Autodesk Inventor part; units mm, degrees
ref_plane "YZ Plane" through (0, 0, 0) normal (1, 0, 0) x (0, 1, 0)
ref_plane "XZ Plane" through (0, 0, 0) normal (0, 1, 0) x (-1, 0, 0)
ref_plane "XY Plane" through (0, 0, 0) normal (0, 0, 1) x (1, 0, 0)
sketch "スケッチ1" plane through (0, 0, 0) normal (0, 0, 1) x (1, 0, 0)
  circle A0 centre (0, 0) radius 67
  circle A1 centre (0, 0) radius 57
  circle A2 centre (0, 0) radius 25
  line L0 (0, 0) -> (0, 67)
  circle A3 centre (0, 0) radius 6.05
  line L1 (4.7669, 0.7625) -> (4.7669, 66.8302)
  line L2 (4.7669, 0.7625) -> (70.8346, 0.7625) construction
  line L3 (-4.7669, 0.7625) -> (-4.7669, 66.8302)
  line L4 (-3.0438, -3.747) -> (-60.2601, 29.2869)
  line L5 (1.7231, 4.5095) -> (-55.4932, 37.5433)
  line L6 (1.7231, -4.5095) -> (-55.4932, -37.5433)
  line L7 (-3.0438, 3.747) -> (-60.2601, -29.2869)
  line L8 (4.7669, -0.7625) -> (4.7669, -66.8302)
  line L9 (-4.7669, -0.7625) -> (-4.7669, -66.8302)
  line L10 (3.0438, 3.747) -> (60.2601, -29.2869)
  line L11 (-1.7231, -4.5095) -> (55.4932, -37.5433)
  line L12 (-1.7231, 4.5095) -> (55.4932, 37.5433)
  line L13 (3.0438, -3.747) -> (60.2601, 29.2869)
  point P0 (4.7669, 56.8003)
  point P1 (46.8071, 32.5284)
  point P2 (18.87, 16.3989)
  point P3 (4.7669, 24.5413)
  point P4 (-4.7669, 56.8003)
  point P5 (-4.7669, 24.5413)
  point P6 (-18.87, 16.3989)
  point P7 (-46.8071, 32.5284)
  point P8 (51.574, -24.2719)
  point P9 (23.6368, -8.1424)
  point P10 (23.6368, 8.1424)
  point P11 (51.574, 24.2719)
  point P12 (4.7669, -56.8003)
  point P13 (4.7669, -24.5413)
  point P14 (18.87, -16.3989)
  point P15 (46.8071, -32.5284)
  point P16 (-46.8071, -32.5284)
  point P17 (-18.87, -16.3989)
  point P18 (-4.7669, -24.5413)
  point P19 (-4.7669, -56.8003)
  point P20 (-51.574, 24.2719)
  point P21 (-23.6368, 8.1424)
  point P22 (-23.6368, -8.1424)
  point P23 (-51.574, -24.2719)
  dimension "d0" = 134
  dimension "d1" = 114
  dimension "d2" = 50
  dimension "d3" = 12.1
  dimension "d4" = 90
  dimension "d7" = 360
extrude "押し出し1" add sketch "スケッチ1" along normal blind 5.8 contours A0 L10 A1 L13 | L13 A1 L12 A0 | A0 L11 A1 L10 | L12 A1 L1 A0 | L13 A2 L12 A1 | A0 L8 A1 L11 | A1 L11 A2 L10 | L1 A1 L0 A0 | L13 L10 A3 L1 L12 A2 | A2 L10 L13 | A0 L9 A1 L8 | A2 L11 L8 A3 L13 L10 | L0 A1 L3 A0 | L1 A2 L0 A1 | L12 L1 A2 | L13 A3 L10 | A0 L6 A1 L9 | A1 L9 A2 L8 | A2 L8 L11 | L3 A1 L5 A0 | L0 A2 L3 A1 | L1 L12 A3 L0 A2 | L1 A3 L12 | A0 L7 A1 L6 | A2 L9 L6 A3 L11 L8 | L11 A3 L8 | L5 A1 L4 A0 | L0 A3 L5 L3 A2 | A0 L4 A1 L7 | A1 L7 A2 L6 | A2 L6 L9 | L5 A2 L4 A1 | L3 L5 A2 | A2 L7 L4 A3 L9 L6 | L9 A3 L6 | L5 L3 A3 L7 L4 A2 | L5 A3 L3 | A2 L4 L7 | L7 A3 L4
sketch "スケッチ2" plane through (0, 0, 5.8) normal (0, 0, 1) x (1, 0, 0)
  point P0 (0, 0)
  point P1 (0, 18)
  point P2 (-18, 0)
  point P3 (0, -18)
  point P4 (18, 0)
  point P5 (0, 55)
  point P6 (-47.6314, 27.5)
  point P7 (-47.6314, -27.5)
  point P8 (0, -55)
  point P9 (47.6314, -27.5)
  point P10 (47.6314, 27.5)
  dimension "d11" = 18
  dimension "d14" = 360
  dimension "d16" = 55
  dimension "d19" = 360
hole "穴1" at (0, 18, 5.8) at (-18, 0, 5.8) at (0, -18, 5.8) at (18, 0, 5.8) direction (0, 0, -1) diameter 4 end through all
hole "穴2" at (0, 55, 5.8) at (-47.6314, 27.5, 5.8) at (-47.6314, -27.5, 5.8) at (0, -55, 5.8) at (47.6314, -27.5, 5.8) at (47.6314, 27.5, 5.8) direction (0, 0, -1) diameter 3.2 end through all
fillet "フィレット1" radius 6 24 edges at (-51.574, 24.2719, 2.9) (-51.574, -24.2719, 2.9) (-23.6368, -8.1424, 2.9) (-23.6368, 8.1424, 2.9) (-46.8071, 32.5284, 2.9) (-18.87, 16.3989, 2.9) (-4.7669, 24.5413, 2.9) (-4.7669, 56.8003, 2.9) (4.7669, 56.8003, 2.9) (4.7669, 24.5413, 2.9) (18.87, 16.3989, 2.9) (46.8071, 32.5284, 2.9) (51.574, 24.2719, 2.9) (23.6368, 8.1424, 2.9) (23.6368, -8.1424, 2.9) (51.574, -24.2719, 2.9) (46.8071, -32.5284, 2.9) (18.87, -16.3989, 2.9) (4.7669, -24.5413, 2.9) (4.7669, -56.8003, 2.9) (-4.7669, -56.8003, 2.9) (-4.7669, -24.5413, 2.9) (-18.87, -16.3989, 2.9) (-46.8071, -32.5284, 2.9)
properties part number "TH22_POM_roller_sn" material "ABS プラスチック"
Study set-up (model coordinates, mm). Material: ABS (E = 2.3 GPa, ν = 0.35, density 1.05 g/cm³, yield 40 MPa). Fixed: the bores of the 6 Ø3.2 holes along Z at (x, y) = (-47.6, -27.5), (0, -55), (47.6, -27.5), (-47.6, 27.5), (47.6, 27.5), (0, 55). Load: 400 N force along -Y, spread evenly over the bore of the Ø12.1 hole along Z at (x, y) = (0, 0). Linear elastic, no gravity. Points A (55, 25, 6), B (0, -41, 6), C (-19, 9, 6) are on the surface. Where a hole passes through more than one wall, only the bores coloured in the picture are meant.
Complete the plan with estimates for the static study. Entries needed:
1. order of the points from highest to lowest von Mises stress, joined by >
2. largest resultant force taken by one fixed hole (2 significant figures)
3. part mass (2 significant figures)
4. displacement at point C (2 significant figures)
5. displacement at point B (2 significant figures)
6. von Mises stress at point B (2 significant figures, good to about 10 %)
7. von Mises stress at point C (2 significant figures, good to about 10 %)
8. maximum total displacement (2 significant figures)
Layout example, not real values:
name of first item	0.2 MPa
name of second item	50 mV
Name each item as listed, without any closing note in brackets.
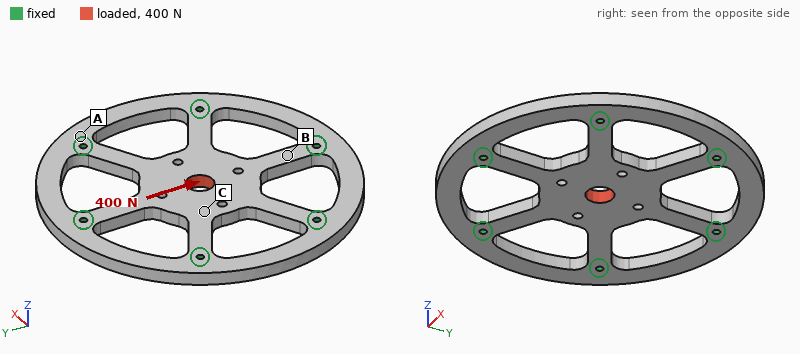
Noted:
order of the points from highest to lowest von Mises stress, joined by >	B > C > A
largest resultant force taken by one fixed hole	120 N
part mass	47 g
displacement at point C	31 µm
displacement at point B	13 µm
von Mises stress at point B	2.3 MPa
von Mises stress at point C	1.1 MPa
maximum total displacement	45 µm
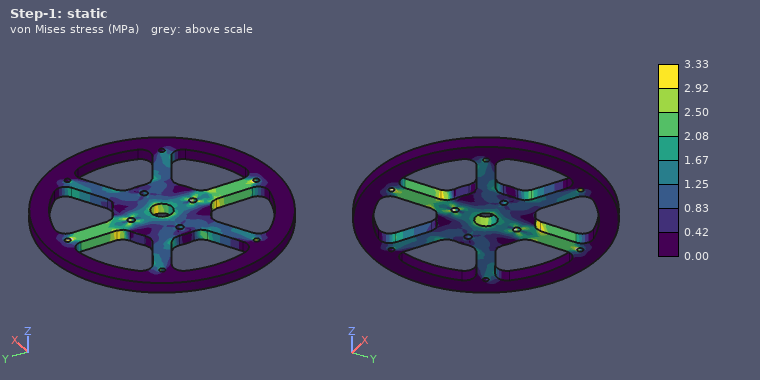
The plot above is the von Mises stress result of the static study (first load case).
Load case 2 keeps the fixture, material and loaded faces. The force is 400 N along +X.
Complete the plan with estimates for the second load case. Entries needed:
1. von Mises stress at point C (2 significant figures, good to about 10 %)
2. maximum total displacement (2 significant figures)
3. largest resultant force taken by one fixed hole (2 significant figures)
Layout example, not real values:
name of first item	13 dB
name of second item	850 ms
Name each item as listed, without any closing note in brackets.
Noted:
von Mises stress at point C	1.5 MPa
maximum total displacement	43 µm
largest resultant force taken by one fixed hole	110 N
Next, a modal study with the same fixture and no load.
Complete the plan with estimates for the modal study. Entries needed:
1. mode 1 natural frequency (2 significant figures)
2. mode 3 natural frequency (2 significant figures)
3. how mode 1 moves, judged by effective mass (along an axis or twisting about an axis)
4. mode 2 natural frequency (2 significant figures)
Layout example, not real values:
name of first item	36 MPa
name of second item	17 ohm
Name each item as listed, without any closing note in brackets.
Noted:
mode 1 natural frequency	870 Hz
mode 3 natural frequency	1800 Hz
how mode 1 moves, judged by effective mass	along Z
mode 2 natural frequency	1700 Hz
